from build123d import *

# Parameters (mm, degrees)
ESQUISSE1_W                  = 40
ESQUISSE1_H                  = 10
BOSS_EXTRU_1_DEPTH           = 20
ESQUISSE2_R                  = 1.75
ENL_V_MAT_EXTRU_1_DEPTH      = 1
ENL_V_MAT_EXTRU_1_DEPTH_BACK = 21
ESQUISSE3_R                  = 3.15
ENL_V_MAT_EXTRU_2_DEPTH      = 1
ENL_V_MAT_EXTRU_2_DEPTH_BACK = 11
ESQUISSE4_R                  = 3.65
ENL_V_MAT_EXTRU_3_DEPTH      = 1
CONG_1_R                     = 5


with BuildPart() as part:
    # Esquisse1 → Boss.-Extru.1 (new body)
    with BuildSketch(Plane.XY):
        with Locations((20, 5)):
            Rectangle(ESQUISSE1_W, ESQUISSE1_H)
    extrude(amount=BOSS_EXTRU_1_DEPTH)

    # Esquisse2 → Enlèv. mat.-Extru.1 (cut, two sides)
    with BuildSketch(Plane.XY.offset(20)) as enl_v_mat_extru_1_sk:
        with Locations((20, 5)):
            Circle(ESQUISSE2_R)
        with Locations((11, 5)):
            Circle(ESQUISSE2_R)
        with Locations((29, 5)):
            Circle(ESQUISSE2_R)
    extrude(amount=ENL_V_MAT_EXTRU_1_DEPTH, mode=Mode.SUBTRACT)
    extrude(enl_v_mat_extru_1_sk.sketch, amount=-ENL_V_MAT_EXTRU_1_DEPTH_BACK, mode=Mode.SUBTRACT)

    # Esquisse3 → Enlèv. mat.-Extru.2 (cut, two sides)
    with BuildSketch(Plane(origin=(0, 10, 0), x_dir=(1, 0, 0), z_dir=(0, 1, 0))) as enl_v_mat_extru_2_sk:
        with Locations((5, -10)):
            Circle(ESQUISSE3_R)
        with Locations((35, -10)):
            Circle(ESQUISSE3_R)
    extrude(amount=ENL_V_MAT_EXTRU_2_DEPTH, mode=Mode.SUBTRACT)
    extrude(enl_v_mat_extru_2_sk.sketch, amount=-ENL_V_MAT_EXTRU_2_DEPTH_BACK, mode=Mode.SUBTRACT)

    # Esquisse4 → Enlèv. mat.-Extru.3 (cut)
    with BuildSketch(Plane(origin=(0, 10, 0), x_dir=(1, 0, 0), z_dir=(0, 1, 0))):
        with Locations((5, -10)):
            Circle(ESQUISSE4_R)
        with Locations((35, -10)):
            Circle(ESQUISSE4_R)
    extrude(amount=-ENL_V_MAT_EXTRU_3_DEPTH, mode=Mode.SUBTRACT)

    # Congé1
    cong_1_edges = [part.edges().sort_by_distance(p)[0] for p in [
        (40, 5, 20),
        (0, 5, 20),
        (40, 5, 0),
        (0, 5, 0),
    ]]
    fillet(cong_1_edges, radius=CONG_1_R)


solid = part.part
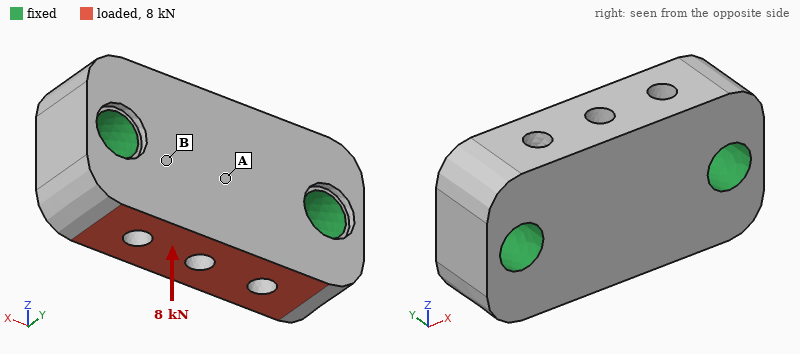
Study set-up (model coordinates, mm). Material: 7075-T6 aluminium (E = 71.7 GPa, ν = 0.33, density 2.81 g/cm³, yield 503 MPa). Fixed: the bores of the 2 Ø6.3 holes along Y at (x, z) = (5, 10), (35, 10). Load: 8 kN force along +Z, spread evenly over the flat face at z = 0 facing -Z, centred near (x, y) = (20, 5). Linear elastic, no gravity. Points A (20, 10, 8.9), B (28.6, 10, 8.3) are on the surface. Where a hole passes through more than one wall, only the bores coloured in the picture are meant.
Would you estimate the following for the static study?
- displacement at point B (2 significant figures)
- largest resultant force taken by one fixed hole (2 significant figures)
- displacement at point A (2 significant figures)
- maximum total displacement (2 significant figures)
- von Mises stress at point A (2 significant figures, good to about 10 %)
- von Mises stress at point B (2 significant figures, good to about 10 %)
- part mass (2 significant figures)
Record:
5.9 µm
4.1 kN
9.8 µm
12 µm
16 MPa
38 MPa
18 g
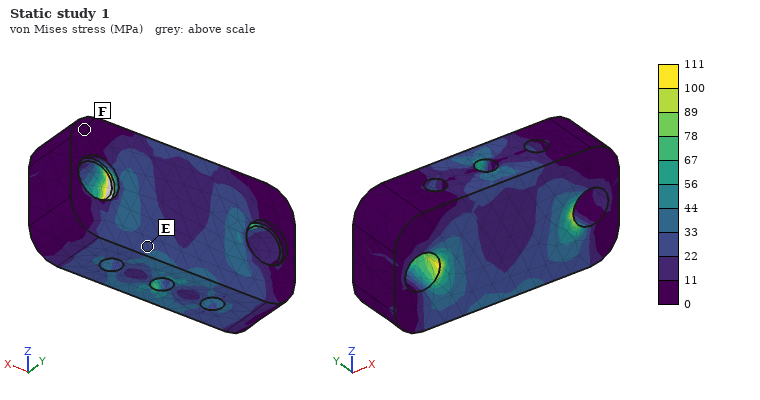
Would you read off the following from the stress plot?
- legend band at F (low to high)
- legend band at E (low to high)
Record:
0 to 11 MPa
22 to 33 MPa
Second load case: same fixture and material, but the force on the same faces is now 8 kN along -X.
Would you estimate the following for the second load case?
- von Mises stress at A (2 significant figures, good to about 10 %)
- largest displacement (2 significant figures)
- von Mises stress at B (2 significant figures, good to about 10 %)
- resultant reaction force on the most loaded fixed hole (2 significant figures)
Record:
25 MPa
13 µm
31 MPa
4.5 kN
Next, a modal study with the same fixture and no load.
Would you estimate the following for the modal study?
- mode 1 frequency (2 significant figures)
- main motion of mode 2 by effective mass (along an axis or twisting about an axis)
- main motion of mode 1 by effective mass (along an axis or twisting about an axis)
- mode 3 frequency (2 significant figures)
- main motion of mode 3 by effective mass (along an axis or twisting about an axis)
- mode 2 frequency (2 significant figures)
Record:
33 kHz
twisting about X
along Y
41 kHz
along Z
37 kHz
